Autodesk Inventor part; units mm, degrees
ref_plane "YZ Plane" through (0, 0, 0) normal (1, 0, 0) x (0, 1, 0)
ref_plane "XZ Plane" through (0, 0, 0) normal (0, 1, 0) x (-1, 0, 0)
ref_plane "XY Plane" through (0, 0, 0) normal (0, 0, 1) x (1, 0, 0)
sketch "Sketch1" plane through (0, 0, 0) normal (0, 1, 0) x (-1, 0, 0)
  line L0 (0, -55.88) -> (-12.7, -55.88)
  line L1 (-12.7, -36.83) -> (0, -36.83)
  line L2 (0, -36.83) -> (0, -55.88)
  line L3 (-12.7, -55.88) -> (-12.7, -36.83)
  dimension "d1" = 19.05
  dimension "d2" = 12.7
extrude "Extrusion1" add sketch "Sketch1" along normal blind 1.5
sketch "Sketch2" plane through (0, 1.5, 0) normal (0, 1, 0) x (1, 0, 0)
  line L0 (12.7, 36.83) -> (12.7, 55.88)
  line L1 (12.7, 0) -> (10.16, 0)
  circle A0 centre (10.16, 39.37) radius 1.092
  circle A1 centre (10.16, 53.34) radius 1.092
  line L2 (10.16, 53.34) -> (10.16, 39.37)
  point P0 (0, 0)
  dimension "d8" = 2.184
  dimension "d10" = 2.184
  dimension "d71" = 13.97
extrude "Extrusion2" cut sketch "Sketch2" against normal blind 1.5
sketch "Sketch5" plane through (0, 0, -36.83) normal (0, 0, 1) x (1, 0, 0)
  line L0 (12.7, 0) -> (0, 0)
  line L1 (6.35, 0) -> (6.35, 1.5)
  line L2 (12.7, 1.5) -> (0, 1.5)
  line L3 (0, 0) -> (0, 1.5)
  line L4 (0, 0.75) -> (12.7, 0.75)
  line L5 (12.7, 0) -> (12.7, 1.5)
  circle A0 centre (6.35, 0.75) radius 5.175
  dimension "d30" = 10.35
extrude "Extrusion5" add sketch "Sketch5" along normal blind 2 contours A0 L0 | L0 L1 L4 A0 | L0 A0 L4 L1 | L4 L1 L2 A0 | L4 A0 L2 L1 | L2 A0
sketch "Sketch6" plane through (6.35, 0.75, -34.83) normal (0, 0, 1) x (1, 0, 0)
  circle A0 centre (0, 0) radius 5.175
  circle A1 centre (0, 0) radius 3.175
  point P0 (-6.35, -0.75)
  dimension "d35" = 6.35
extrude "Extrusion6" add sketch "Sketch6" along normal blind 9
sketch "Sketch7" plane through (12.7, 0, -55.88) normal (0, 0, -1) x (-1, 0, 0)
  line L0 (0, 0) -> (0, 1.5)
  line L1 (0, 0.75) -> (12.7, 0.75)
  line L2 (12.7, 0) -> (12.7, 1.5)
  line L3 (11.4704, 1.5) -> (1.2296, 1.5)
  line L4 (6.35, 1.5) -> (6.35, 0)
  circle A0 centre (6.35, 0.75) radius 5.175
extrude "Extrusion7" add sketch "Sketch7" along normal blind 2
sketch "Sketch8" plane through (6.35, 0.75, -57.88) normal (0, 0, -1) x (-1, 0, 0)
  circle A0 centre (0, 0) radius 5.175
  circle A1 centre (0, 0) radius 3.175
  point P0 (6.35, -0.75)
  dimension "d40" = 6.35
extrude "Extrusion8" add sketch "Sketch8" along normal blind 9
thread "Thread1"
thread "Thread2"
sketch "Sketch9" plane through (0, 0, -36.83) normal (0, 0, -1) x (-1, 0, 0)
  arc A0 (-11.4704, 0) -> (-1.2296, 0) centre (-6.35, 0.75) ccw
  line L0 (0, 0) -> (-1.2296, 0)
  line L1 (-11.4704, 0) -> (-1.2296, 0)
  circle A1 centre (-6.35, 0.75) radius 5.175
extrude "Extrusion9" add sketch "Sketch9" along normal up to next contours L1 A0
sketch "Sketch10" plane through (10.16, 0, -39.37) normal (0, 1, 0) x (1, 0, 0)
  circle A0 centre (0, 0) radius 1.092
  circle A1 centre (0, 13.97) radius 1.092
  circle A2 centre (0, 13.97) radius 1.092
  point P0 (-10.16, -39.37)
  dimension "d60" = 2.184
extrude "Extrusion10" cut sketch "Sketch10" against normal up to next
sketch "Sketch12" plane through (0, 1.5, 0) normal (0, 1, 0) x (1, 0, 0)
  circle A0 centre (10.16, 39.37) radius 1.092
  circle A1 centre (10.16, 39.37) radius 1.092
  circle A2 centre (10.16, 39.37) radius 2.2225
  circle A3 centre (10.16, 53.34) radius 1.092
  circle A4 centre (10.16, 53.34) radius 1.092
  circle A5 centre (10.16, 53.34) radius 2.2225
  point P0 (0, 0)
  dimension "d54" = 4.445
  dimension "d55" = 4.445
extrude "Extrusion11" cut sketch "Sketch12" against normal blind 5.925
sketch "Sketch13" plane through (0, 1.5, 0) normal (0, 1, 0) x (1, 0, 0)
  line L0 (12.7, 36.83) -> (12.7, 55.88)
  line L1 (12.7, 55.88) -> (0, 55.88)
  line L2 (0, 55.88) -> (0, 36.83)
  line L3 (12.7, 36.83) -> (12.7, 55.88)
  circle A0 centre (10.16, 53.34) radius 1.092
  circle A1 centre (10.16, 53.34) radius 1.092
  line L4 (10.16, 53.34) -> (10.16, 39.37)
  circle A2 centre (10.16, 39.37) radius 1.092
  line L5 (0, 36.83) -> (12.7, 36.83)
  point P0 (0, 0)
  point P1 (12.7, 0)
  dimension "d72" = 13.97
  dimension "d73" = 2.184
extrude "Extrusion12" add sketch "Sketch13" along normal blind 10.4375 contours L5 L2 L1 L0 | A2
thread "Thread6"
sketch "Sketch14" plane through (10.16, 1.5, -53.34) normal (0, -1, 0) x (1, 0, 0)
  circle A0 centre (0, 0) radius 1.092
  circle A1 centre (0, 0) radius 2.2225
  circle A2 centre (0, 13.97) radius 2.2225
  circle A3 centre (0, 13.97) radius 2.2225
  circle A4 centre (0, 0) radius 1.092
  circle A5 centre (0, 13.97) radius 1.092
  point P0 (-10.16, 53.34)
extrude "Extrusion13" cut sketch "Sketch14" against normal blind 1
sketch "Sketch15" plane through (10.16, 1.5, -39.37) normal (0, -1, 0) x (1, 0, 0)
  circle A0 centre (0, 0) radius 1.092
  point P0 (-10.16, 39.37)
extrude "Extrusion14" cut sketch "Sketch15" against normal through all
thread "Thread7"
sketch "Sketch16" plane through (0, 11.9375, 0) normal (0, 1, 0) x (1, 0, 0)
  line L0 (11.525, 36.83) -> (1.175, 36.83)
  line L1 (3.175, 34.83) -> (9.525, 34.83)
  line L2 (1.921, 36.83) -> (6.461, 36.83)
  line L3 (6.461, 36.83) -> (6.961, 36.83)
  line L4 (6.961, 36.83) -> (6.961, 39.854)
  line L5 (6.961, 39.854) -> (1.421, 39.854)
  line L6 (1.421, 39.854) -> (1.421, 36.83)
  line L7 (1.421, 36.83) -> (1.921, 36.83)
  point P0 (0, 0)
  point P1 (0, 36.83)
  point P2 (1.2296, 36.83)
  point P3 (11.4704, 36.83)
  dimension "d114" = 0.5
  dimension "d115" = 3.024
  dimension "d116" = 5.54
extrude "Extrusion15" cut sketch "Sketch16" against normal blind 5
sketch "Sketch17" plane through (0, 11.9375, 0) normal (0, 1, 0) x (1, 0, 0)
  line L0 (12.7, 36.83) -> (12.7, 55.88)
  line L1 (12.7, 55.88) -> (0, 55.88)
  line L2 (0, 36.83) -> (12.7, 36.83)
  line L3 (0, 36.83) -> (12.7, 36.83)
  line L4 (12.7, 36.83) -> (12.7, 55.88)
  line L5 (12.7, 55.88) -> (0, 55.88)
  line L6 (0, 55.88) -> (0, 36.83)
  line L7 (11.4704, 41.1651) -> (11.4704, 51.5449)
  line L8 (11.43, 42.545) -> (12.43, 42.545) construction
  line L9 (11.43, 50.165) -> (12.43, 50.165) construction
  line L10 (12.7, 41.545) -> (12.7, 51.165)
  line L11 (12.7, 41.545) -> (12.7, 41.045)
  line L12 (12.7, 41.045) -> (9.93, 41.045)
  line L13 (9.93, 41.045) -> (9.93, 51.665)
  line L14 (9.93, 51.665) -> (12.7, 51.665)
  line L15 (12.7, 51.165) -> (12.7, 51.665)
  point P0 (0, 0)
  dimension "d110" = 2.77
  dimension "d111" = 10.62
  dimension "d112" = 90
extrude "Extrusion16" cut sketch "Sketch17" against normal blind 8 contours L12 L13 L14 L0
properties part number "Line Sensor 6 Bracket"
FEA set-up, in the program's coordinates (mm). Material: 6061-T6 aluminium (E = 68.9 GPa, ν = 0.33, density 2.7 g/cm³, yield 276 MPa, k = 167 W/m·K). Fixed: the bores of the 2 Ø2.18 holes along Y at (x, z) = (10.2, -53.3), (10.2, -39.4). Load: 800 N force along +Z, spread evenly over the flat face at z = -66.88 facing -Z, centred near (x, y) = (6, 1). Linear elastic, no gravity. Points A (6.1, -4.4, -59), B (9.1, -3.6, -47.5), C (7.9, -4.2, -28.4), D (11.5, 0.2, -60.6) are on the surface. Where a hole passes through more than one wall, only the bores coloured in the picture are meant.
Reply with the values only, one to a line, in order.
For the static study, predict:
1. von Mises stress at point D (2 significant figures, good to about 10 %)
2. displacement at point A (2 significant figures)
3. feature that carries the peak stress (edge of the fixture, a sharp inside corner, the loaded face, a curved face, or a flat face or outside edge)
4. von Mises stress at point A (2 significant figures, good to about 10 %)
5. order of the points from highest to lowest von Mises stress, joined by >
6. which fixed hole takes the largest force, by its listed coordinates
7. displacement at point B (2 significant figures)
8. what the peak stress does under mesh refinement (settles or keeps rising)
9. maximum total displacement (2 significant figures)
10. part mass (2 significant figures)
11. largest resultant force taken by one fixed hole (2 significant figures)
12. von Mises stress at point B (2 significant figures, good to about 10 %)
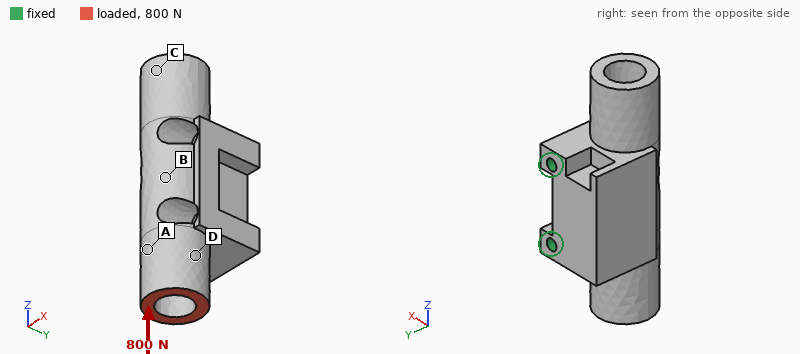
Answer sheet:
13 MPa
5.2 µm
edge of the fixture
17 MPa
A > D > B > C
(10.2, -53.3)
1.8 µm
keeps rising
8.1 µm
12 g
580 N
6.8 MPa
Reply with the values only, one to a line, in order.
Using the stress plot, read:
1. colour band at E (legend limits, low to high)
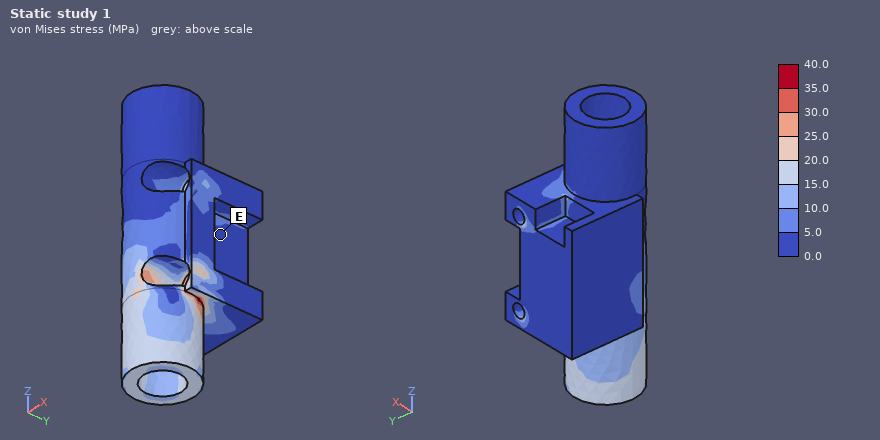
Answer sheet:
0.0 to 5.0 MPa
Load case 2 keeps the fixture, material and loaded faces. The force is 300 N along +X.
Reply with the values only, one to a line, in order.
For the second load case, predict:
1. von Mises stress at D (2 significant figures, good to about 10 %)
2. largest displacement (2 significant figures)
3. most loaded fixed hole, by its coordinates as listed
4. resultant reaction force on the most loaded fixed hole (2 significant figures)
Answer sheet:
17 MPa
20 µm
(10.2, -53.3)
580 N
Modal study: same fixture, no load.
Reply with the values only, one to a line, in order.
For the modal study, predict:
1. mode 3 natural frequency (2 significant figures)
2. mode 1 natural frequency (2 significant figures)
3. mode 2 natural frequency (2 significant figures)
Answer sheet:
24 kHz
21 kHz
22 kHz
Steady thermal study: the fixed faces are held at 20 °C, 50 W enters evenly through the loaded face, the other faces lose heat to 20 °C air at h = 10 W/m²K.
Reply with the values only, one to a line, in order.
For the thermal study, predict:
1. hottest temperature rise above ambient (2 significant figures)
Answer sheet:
83 K
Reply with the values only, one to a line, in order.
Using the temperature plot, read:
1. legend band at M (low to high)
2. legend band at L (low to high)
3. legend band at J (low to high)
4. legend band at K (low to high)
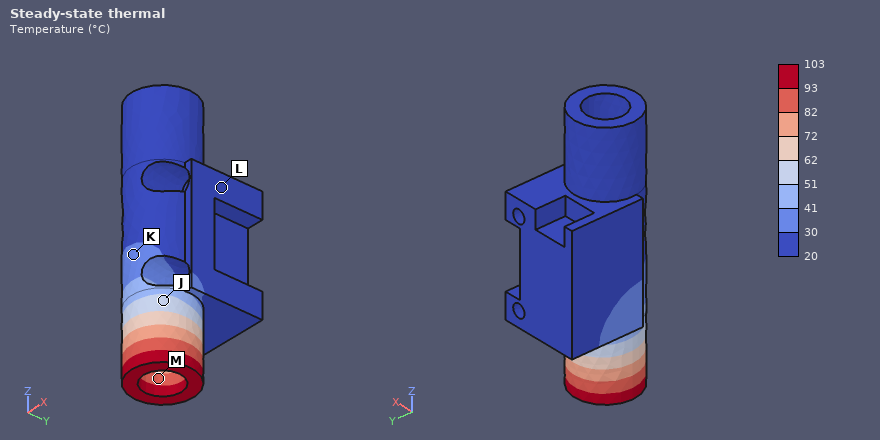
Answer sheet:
82 to 93 °C
20 to 30 °C
51 to 62 °C
30 to 41 °C
